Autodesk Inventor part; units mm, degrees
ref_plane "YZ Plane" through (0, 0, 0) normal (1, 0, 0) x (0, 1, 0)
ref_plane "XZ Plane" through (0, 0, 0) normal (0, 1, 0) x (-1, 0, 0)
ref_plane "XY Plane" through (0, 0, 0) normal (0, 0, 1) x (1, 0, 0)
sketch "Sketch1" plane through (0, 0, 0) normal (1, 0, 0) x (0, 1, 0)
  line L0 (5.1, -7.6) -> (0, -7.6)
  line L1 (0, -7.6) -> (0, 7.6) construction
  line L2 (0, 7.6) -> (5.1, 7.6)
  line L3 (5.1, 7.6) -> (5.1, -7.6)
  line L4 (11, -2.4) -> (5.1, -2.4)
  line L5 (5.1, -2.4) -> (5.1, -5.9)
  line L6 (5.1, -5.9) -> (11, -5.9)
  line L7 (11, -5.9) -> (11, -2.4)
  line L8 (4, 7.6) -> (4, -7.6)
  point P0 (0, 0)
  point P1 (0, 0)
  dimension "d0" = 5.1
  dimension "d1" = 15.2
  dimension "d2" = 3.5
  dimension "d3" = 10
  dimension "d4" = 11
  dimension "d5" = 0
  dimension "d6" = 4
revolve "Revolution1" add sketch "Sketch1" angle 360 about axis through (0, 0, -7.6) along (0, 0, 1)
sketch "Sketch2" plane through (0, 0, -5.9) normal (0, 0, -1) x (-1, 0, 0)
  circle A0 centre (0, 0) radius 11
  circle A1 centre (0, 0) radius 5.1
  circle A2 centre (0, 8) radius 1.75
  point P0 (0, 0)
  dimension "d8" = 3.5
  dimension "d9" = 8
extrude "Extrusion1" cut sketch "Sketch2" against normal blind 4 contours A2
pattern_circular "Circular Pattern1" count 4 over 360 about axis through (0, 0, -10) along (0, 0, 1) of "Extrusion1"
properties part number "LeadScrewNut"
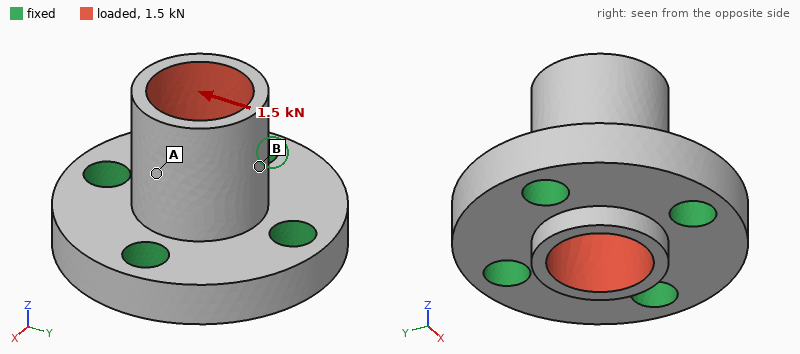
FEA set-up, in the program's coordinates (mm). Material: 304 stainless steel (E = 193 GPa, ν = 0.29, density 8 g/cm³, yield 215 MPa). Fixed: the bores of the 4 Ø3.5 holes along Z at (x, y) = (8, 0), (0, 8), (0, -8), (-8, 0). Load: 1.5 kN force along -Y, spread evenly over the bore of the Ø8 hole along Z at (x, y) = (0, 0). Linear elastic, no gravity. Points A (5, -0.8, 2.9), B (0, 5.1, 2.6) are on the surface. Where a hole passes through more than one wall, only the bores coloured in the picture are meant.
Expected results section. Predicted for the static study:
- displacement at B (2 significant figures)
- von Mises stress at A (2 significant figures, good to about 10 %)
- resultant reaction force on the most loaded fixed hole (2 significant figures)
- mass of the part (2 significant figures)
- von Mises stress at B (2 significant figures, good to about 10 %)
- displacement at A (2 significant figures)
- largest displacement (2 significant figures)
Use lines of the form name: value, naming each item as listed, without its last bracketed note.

displacement at B: 6.0 µm
von Mises stress at A: 47 MPa
resultant reaction force on the most loaded fixed hole: 610 N
mass of the part: 11 g
von Mises stress at B: 22 MPa
displacement at A: 5.3 µm
largest displacement: 9.1 µm
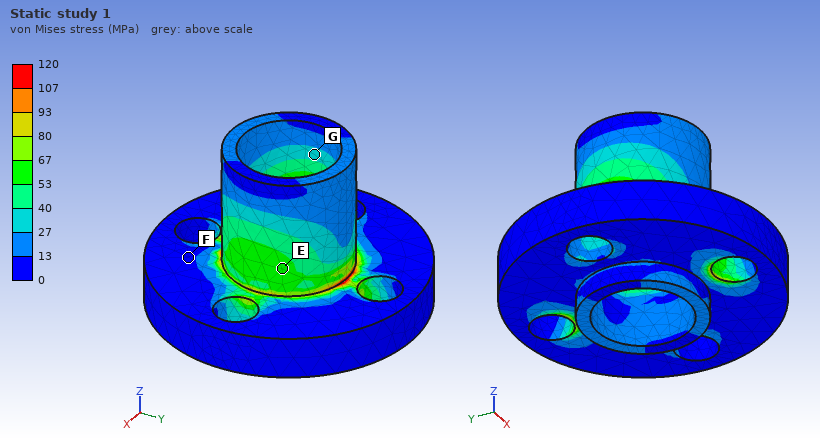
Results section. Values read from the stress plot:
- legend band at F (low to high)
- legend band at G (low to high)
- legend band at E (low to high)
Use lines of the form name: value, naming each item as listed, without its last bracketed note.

legend band at F: 0 to 13 MPa
legend band at G: 27 to 40 MPa
legend band at E: 53 to 67 MPa
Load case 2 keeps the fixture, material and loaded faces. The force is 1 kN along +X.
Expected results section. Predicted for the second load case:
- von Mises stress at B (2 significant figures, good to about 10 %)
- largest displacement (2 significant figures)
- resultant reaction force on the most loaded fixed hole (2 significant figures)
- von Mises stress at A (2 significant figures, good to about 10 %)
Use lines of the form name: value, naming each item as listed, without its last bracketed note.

von Mises stress at B: 33 MPa
largest displacement: 6.1 µm
resultant reaction force on the most loaded fixed hole: 410 N
von Mises stress at A: 15 MPa
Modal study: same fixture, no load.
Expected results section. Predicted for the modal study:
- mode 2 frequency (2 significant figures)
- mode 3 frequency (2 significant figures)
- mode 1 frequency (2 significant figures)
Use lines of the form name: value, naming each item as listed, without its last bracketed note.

mode 2 frequency: 38 kHz
mode 3 frequency: 40 kHz
mode 1 frequency: 38 kHz
